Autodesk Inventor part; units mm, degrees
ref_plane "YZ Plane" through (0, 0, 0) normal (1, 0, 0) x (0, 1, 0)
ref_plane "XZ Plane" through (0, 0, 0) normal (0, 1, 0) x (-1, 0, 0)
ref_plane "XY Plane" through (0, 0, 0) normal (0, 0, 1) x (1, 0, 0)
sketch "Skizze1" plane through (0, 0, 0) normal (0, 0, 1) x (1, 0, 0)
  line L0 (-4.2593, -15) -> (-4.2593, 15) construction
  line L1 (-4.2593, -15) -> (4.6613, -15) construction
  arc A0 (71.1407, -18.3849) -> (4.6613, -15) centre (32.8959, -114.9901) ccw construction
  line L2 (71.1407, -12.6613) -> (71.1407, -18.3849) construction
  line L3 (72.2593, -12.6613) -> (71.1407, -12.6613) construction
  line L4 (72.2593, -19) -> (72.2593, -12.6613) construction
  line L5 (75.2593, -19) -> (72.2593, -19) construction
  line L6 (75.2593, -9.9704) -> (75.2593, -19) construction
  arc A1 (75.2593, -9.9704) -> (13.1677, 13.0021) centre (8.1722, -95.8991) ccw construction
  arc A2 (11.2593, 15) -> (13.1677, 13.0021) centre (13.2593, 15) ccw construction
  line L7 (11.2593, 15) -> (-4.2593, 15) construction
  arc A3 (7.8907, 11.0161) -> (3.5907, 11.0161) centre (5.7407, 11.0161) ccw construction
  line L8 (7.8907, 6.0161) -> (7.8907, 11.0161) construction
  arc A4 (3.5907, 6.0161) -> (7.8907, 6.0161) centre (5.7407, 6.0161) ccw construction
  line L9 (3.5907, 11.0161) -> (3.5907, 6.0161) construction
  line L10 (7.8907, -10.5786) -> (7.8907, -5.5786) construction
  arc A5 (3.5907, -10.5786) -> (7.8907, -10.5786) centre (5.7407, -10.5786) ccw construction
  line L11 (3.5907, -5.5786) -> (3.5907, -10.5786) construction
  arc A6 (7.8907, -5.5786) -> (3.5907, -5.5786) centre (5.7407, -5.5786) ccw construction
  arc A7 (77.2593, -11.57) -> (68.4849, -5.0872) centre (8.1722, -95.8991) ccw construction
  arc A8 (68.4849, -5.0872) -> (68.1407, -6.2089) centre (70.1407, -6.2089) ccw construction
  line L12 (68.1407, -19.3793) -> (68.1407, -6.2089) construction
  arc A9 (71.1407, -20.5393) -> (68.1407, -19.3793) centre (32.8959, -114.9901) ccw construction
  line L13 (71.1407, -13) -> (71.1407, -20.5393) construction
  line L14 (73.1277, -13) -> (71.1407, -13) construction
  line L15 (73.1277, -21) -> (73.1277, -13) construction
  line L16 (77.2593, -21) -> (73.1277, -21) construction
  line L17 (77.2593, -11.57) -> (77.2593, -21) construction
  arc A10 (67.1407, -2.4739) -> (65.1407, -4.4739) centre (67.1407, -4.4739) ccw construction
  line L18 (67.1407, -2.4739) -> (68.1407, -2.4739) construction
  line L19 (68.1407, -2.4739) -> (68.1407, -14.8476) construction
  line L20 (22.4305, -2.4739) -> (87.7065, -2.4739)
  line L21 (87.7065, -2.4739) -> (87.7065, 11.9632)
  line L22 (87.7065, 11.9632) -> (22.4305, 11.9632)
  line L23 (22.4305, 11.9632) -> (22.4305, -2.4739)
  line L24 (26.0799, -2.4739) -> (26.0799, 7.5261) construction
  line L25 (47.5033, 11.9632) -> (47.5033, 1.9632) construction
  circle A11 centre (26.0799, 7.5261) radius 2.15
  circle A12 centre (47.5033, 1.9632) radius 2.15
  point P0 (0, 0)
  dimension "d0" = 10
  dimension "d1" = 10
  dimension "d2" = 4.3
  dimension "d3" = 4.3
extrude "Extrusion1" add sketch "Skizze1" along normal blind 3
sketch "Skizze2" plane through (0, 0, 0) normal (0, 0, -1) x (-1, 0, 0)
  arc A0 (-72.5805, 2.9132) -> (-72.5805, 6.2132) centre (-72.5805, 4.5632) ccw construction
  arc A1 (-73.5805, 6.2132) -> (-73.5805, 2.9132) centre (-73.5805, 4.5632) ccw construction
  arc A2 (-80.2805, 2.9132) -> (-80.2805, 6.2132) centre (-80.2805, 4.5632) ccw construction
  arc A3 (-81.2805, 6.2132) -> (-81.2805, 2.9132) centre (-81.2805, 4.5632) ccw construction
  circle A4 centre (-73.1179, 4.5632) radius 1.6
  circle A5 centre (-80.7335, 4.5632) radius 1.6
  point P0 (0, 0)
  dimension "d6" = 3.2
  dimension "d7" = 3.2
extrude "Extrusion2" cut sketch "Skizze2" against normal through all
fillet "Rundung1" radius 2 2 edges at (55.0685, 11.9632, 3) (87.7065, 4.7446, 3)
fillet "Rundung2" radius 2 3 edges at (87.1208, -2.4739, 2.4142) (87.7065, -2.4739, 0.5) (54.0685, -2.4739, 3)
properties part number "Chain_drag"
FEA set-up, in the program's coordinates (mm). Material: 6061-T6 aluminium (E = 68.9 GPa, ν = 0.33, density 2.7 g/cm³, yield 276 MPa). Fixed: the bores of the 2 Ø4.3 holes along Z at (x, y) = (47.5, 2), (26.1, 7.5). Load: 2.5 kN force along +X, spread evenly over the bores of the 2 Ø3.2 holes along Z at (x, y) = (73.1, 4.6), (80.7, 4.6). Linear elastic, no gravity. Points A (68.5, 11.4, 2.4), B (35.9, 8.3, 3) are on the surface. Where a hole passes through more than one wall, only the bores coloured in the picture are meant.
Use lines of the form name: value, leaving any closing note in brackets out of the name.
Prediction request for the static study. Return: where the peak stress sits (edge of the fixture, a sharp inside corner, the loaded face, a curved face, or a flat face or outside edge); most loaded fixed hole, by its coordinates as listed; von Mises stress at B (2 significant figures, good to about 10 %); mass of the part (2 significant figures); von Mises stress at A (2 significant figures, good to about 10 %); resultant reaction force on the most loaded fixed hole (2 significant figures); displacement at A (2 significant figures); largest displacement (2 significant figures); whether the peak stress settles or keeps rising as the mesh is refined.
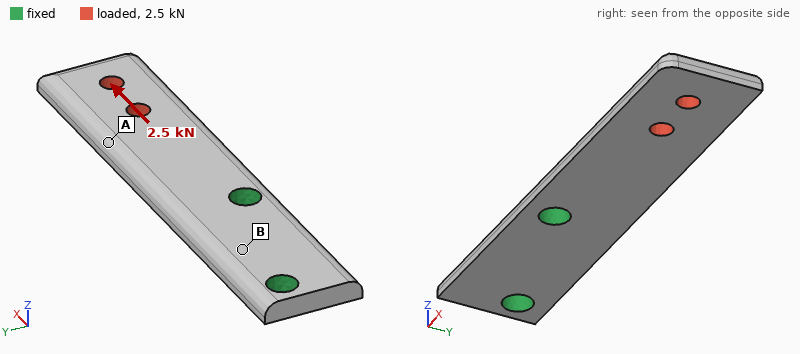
where the peak stress sits: edge of the fixture
most loaded fixed hole, by its coordinates as listed: (47.5, 2)
von Mises stress at B: 19 MPa
mass of the part: 6.9 g
von Mises stress at A: 56 MPa
resultant reaction force on the most loaded fixed hole: 2.2 kN
displacement at A: 32 µm
largest displacement: 53 µm
whether the peak stress settles or keeps rising as the mesh is refined: keeps rising
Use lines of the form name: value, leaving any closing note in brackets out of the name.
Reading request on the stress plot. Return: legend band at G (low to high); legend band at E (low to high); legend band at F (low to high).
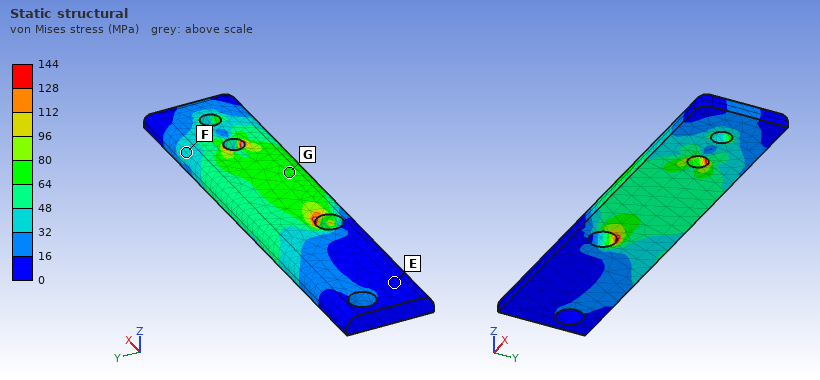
legend band at G: 64 to 80 MPa
legend band at E: 0 to 16 MPa
legend band at F: 32 to 48 MPa
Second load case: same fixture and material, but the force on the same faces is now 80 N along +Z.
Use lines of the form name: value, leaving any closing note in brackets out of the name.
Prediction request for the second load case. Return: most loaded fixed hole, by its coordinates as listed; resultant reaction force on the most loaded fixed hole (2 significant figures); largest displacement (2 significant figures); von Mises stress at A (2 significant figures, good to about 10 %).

most loaded fixed hole, by its coordinates as listed: (47.5, 2)
resultant reaction force on the most loaded fixed hole: 95 N
largest displacement: 0.48 mm
von Mises stress at A: 23 MPa
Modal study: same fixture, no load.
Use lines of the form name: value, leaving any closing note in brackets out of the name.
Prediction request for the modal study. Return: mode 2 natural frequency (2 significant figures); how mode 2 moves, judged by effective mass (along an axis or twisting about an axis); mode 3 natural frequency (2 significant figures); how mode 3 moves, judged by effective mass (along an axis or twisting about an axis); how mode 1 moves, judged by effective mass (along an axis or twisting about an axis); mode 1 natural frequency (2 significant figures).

mode 2 natural frequency: 5800 Hz
how mode 2 moves, judged by effective mass: along Y
mode 3 natural frequency: 7800 Hz
how mode 3 moves, judged by effective mass: twisting about X
how mode 1 moves, judged by effective mass: along Z
mode 1 natural frequency: 1600 Hz
